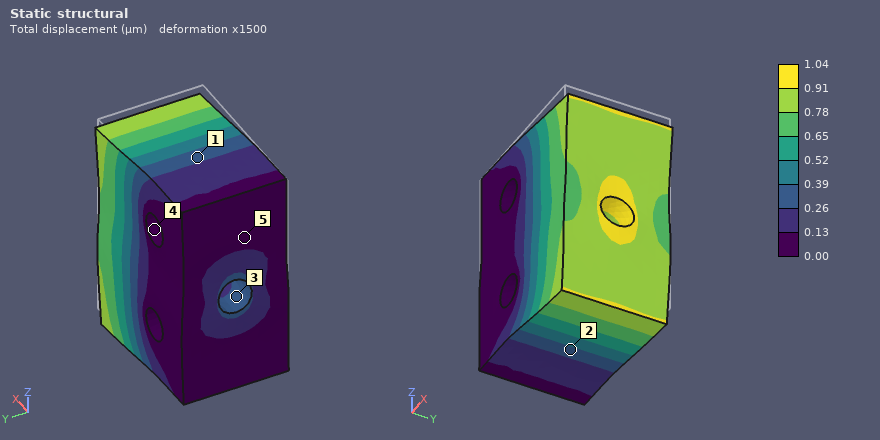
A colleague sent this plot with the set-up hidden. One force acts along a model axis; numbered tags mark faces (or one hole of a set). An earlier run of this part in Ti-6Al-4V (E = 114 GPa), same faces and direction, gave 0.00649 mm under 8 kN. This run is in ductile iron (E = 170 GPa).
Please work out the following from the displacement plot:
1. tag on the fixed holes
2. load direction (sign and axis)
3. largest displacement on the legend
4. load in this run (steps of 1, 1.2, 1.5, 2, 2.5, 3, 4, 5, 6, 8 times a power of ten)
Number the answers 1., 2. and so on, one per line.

1. 4
2. -Z
3. 1.04 µm
4. 2 kN
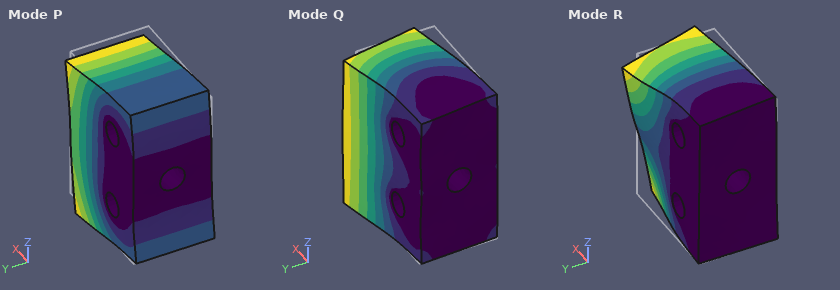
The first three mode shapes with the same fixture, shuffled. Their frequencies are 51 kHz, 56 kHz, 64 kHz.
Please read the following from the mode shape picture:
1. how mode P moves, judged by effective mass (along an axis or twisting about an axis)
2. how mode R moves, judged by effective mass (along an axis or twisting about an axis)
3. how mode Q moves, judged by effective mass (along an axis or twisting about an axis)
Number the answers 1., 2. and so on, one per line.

1. along Z
2. twisting about X
3. along Y
